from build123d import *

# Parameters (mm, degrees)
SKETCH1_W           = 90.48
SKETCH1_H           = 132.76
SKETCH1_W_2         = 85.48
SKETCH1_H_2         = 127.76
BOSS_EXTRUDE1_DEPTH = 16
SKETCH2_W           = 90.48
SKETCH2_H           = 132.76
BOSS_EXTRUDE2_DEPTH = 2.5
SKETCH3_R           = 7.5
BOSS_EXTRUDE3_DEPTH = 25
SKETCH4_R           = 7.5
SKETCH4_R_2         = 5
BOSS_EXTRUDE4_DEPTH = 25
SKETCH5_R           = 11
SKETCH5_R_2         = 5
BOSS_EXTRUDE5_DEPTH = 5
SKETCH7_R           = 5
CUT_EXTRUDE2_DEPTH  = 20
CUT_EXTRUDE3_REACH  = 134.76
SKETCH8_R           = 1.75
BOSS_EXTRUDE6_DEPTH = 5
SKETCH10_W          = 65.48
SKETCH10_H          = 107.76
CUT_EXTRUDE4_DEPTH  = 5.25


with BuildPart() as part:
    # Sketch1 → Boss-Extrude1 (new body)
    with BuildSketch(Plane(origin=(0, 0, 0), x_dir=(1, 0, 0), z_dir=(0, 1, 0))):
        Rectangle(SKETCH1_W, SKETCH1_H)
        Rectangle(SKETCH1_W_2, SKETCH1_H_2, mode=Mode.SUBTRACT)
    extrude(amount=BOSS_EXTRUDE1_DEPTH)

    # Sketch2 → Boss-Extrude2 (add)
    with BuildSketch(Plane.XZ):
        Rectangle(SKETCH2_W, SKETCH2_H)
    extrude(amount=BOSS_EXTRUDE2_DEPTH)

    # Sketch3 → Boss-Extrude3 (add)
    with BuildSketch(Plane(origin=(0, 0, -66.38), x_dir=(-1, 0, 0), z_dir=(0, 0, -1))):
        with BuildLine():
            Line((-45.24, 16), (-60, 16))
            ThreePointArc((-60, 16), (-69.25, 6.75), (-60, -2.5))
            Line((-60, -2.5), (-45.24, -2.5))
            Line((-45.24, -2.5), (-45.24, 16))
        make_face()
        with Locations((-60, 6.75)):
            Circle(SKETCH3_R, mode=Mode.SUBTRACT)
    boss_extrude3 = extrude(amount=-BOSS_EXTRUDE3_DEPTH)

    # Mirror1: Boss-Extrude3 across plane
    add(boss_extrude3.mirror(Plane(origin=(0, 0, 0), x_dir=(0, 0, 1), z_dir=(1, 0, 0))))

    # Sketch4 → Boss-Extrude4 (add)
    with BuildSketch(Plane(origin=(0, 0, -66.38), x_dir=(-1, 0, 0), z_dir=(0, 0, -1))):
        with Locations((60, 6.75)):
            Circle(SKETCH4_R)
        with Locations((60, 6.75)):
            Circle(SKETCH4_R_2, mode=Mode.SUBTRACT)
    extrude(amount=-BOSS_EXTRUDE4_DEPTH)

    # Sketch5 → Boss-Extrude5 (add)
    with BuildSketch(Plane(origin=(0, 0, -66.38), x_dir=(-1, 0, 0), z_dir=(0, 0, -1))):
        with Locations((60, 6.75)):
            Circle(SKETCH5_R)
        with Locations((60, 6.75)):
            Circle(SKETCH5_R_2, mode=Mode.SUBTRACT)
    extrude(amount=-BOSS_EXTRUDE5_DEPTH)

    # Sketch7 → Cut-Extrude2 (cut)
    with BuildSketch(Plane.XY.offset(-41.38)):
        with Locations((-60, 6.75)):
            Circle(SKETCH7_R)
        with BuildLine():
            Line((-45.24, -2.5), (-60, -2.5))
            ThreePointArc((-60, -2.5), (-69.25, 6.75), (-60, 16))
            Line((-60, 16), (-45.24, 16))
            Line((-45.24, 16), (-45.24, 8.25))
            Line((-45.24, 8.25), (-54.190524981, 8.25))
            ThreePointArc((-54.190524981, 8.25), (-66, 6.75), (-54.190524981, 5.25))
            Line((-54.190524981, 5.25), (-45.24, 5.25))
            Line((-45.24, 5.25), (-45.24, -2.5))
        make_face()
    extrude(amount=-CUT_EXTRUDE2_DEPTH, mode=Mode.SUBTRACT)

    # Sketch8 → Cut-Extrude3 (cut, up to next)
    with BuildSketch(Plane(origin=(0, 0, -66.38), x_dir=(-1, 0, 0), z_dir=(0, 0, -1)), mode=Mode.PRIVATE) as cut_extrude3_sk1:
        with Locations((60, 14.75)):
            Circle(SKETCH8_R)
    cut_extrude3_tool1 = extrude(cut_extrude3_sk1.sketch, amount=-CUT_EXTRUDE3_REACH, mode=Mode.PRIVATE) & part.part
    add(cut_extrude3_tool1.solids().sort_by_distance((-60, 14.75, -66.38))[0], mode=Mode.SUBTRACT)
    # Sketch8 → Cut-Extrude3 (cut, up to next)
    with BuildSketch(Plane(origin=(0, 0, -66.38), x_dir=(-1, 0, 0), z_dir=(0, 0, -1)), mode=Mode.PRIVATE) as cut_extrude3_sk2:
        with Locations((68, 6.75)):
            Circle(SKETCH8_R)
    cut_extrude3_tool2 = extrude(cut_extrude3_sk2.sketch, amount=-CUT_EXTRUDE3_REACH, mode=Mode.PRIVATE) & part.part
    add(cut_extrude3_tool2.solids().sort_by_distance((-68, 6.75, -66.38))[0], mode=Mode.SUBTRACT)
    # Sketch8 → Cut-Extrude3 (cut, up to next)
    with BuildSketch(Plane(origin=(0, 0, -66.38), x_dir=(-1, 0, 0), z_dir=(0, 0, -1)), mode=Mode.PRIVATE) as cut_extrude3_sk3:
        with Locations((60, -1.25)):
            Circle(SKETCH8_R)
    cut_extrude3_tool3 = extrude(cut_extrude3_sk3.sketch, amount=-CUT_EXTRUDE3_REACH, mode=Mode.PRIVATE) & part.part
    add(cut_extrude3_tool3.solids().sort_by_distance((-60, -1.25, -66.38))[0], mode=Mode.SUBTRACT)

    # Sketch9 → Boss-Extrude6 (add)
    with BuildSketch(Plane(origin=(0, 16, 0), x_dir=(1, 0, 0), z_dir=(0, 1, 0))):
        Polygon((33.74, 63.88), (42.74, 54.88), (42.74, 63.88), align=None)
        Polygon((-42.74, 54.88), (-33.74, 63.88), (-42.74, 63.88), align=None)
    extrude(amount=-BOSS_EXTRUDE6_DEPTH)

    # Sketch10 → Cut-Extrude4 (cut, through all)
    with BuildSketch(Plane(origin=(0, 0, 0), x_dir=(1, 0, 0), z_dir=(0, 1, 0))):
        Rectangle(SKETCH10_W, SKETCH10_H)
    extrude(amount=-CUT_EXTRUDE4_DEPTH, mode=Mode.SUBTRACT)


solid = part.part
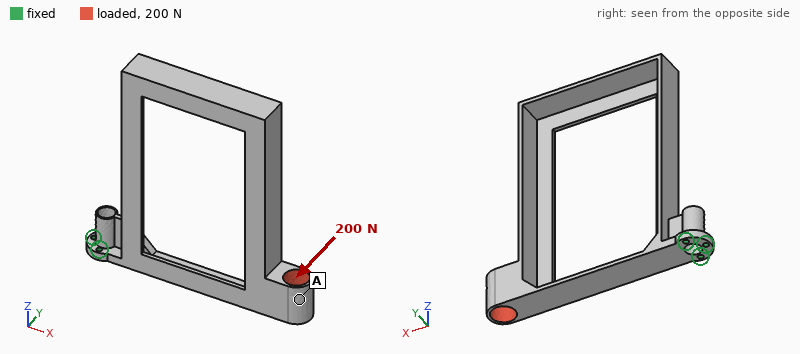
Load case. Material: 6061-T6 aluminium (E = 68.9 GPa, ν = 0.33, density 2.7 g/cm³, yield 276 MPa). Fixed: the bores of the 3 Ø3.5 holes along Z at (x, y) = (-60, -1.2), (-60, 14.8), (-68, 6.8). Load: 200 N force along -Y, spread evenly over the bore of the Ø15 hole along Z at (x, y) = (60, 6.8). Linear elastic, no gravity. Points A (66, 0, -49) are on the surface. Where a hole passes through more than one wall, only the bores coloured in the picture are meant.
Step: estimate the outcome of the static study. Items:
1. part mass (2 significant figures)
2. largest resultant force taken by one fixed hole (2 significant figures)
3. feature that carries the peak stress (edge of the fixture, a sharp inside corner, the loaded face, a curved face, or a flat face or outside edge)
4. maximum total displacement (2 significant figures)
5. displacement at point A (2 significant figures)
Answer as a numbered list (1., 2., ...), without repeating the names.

1. 110 g
2. 1.5 kN
3. a flat face or outside edge
4. 1.8 mm
5. 0.98 mm
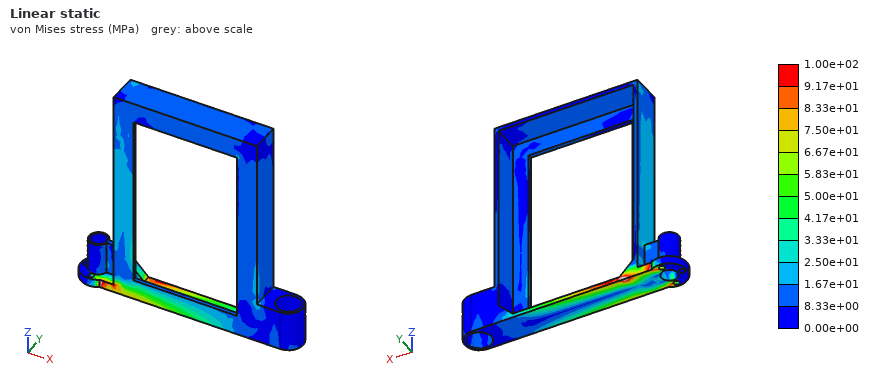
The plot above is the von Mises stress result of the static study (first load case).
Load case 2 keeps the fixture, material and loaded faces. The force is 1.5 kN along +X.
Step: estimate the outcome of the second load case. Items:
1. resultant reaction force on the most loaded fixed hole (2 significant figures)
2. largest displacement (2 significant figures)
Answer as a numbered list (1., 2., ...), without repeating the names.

1. 750 N
2. 2.1 mm
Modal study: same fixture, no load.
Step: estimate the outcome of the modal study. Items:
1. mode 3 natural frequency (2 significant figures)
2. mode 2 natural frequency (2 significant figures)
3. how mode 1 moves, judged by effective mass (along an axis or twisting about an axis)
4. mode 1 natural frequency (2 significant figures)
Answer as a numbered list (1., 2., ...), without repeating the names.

1. 510 Hz
2. 180 Hz
3. along Y
4. 150 Hz
